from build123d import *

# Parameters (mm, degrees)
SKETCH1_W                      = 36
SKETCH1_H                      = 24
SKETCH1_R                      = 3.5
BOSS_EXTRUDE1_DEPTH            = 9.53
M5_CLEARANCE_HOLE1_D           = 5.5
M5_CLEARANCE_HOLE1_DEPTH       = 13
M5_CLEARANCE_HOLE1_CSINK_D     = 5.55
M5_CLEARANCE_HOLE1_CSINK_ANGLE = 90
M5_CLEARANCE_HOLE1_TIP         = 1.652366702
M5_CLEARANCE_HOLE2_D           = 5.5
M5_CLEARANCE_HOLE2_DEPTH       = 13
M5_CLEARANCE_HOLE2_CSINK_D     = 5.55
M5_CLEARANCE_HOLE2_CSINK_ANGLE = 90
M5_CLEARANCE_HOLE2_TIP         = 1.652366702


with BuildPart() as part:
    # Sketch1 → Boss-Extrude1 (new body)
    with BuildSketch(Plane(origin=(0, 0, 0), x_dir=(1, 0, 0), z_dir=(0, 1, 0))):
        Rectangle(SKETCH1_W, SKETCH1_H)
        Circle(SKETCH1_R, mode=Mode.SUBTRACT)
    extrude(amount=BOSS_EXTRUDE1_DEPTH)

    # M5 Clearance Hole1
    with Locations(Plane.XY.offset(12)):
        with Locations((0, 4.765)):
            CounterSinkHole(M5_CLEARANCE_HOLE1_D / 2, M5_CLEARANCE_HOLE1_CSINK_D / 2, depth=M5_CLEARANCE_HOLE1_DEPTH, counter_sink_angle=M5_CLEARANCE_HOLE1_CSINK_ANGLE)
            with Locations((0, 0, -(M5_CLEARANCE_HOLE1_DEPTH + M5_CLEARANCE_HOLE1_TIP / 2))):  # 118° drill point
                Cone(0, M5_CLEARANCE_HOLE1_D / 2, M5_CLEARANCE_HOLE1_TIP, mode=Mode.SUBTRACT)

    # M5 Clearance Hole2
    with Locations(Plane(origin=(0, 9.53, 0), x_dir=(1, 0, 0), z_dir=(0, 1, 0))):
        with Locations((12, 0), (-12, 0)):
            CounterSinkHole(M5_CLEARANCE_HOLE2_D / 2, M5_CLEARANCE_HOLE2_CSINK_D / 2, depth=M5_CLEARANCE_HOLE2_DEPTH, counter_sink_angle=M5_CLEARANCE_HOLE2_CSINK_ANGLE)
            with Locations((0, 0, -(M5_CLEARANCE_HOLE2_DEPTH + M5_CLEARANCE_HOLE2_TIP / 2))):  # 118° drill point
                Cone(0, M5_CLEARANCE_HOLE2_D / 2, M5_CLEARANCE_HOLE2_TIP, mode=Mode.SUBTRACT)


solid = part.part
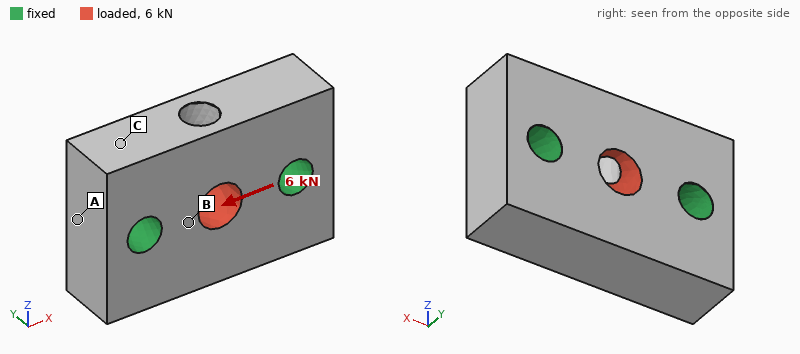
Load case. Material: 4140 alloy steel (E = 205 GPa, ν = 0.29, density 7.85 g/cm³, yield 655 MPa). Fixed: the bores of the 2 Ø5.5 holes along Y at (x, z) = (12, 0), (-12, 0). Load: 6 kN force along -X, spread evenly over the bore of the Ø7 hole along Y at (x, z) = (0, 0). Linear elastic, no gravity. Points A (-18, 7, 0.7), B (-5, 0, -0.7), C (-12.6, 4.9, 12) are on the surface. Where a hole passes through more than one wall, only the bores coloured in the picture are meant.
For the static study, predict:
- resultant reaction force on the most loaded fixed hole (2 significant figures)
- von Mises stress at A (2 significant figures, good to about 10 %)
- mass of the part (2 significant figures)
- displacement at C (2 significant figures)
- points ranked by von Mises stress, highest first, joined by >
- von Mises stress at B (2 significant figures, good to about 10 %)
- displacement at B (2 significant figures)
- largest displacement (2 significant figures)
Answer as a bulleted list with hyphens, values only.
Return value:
- 3.0 kN
- 9.5 MPa
- 57 g
- 0.50 µm
- B > A > C
- 39 MPa
- 0.88 µm
- 1.6 µm
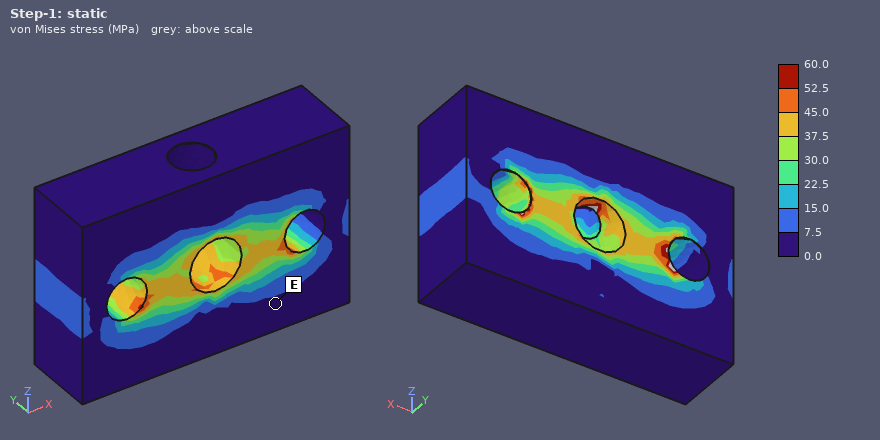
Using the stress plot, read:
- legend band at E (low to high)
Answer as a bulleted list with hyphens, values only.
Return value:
- 0.0 to 7.5 MPa
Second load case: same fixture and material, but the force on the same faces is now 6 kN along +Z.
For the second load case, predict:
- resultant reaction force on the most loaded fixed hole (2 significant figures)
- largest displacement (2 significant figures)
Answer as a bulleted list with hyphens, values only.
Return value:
- 3.0 kN
- 2.8 µm
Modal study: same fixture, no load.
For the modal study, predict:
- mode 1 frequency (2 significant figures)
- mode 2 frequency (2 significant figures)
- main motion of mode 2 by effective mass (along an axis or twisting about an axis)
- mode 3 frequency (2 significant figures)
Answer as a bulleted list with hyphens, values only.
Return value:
- 36 kHz
- 41 kHz
- along Y
- 50 kHz
